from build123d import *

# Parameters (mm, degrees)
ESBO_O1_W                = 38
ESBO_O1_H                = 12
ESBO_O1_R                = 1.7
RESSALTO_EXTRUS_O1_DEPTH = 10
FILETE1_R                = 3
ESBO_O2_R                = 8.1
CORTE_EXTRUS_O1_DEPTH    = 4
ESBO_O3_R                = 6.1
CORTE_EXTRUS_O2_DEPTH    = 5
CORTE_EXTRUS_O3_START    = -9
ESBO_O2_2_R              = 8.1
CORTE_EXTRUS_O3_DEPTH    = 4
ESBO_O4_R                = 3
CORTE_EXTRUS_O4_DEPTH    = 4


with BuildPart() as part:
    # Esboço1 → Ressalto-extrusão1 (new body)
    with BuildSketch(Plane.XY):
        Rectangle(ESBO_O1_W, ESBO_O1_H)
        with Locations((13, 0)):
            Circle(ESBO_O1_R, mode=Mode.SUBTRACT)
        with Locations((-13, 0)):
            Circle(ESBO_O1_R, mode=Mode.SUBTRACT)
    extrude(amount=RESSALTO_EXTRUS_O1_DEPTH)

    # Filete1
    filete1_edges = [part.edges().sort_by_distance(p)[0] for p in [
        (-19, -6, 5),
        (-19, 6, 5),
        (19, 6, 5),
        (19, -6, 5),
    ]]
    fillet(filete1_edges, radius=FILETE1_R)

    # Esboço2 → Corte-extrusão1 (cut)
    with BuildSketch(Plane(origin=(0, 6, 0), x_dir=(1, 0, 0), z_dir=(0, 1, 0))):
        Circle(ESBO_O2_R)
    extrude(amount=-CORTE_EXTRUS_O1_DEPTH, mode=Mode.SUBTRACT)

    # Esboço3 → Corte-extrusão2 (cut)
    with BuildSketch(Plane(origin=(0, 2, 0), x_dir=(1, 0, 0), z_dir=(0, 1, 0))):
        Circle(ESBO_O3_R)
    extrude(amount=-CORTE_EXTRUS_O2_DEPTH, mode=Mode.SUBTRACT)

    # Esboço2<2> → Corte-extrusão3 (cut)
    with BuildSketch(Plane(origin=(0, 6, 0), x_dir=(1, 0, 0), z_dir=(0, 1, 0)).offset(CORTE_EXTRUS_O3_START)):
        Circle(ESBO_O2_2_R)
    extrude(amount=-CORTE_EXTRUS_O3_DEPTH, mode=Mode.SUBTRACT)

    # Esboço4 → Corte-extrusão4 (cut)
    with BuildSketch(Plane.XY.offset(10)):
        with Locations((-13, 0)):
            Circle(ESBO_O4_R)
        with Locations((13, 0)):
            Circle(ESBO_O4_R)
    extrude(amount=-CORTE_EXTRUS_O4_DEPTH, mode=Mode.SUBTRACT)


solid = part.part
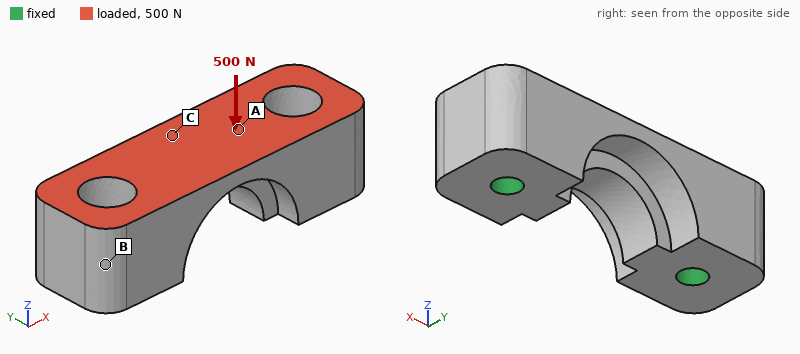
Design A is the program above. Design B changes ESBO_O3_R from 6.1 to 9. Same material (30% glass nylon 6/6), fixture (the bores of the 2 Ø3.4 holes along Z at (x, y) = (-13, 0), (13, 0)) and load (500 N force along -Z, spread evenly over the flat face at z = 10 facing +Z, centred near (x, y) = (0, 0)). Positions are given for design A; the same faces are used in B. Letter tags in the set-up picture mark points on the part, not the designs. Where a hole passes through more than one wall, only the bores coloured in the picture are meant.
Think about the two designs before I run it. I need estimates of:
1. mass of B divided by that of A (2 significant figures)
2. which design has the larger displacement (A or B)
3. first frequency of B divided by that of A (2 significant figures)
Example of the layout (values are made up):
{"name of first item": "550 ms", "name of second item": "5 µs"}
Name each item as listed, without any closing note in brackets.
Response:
{"mass of B divided by that of A": "0.89", "which design has the larger displacement": "B", "first frequency of B divided by that of A": "1.1"}
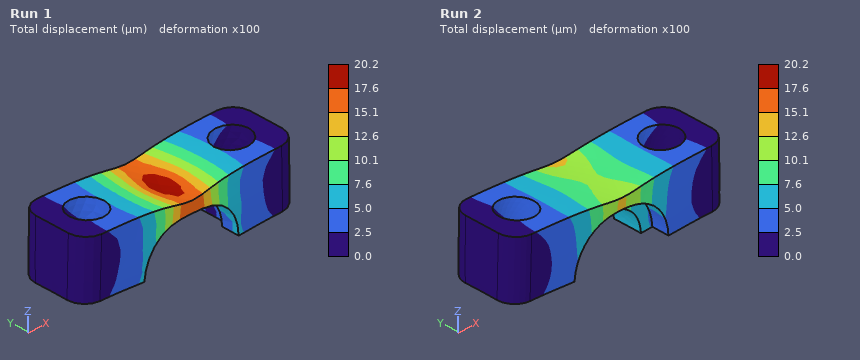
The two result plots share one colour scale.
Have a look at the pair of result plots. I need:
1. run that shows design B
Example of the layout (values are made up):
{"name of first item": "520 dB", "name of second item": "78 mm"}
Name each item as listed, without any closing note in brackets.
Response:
{"run that shows design B": "Run 1"}
